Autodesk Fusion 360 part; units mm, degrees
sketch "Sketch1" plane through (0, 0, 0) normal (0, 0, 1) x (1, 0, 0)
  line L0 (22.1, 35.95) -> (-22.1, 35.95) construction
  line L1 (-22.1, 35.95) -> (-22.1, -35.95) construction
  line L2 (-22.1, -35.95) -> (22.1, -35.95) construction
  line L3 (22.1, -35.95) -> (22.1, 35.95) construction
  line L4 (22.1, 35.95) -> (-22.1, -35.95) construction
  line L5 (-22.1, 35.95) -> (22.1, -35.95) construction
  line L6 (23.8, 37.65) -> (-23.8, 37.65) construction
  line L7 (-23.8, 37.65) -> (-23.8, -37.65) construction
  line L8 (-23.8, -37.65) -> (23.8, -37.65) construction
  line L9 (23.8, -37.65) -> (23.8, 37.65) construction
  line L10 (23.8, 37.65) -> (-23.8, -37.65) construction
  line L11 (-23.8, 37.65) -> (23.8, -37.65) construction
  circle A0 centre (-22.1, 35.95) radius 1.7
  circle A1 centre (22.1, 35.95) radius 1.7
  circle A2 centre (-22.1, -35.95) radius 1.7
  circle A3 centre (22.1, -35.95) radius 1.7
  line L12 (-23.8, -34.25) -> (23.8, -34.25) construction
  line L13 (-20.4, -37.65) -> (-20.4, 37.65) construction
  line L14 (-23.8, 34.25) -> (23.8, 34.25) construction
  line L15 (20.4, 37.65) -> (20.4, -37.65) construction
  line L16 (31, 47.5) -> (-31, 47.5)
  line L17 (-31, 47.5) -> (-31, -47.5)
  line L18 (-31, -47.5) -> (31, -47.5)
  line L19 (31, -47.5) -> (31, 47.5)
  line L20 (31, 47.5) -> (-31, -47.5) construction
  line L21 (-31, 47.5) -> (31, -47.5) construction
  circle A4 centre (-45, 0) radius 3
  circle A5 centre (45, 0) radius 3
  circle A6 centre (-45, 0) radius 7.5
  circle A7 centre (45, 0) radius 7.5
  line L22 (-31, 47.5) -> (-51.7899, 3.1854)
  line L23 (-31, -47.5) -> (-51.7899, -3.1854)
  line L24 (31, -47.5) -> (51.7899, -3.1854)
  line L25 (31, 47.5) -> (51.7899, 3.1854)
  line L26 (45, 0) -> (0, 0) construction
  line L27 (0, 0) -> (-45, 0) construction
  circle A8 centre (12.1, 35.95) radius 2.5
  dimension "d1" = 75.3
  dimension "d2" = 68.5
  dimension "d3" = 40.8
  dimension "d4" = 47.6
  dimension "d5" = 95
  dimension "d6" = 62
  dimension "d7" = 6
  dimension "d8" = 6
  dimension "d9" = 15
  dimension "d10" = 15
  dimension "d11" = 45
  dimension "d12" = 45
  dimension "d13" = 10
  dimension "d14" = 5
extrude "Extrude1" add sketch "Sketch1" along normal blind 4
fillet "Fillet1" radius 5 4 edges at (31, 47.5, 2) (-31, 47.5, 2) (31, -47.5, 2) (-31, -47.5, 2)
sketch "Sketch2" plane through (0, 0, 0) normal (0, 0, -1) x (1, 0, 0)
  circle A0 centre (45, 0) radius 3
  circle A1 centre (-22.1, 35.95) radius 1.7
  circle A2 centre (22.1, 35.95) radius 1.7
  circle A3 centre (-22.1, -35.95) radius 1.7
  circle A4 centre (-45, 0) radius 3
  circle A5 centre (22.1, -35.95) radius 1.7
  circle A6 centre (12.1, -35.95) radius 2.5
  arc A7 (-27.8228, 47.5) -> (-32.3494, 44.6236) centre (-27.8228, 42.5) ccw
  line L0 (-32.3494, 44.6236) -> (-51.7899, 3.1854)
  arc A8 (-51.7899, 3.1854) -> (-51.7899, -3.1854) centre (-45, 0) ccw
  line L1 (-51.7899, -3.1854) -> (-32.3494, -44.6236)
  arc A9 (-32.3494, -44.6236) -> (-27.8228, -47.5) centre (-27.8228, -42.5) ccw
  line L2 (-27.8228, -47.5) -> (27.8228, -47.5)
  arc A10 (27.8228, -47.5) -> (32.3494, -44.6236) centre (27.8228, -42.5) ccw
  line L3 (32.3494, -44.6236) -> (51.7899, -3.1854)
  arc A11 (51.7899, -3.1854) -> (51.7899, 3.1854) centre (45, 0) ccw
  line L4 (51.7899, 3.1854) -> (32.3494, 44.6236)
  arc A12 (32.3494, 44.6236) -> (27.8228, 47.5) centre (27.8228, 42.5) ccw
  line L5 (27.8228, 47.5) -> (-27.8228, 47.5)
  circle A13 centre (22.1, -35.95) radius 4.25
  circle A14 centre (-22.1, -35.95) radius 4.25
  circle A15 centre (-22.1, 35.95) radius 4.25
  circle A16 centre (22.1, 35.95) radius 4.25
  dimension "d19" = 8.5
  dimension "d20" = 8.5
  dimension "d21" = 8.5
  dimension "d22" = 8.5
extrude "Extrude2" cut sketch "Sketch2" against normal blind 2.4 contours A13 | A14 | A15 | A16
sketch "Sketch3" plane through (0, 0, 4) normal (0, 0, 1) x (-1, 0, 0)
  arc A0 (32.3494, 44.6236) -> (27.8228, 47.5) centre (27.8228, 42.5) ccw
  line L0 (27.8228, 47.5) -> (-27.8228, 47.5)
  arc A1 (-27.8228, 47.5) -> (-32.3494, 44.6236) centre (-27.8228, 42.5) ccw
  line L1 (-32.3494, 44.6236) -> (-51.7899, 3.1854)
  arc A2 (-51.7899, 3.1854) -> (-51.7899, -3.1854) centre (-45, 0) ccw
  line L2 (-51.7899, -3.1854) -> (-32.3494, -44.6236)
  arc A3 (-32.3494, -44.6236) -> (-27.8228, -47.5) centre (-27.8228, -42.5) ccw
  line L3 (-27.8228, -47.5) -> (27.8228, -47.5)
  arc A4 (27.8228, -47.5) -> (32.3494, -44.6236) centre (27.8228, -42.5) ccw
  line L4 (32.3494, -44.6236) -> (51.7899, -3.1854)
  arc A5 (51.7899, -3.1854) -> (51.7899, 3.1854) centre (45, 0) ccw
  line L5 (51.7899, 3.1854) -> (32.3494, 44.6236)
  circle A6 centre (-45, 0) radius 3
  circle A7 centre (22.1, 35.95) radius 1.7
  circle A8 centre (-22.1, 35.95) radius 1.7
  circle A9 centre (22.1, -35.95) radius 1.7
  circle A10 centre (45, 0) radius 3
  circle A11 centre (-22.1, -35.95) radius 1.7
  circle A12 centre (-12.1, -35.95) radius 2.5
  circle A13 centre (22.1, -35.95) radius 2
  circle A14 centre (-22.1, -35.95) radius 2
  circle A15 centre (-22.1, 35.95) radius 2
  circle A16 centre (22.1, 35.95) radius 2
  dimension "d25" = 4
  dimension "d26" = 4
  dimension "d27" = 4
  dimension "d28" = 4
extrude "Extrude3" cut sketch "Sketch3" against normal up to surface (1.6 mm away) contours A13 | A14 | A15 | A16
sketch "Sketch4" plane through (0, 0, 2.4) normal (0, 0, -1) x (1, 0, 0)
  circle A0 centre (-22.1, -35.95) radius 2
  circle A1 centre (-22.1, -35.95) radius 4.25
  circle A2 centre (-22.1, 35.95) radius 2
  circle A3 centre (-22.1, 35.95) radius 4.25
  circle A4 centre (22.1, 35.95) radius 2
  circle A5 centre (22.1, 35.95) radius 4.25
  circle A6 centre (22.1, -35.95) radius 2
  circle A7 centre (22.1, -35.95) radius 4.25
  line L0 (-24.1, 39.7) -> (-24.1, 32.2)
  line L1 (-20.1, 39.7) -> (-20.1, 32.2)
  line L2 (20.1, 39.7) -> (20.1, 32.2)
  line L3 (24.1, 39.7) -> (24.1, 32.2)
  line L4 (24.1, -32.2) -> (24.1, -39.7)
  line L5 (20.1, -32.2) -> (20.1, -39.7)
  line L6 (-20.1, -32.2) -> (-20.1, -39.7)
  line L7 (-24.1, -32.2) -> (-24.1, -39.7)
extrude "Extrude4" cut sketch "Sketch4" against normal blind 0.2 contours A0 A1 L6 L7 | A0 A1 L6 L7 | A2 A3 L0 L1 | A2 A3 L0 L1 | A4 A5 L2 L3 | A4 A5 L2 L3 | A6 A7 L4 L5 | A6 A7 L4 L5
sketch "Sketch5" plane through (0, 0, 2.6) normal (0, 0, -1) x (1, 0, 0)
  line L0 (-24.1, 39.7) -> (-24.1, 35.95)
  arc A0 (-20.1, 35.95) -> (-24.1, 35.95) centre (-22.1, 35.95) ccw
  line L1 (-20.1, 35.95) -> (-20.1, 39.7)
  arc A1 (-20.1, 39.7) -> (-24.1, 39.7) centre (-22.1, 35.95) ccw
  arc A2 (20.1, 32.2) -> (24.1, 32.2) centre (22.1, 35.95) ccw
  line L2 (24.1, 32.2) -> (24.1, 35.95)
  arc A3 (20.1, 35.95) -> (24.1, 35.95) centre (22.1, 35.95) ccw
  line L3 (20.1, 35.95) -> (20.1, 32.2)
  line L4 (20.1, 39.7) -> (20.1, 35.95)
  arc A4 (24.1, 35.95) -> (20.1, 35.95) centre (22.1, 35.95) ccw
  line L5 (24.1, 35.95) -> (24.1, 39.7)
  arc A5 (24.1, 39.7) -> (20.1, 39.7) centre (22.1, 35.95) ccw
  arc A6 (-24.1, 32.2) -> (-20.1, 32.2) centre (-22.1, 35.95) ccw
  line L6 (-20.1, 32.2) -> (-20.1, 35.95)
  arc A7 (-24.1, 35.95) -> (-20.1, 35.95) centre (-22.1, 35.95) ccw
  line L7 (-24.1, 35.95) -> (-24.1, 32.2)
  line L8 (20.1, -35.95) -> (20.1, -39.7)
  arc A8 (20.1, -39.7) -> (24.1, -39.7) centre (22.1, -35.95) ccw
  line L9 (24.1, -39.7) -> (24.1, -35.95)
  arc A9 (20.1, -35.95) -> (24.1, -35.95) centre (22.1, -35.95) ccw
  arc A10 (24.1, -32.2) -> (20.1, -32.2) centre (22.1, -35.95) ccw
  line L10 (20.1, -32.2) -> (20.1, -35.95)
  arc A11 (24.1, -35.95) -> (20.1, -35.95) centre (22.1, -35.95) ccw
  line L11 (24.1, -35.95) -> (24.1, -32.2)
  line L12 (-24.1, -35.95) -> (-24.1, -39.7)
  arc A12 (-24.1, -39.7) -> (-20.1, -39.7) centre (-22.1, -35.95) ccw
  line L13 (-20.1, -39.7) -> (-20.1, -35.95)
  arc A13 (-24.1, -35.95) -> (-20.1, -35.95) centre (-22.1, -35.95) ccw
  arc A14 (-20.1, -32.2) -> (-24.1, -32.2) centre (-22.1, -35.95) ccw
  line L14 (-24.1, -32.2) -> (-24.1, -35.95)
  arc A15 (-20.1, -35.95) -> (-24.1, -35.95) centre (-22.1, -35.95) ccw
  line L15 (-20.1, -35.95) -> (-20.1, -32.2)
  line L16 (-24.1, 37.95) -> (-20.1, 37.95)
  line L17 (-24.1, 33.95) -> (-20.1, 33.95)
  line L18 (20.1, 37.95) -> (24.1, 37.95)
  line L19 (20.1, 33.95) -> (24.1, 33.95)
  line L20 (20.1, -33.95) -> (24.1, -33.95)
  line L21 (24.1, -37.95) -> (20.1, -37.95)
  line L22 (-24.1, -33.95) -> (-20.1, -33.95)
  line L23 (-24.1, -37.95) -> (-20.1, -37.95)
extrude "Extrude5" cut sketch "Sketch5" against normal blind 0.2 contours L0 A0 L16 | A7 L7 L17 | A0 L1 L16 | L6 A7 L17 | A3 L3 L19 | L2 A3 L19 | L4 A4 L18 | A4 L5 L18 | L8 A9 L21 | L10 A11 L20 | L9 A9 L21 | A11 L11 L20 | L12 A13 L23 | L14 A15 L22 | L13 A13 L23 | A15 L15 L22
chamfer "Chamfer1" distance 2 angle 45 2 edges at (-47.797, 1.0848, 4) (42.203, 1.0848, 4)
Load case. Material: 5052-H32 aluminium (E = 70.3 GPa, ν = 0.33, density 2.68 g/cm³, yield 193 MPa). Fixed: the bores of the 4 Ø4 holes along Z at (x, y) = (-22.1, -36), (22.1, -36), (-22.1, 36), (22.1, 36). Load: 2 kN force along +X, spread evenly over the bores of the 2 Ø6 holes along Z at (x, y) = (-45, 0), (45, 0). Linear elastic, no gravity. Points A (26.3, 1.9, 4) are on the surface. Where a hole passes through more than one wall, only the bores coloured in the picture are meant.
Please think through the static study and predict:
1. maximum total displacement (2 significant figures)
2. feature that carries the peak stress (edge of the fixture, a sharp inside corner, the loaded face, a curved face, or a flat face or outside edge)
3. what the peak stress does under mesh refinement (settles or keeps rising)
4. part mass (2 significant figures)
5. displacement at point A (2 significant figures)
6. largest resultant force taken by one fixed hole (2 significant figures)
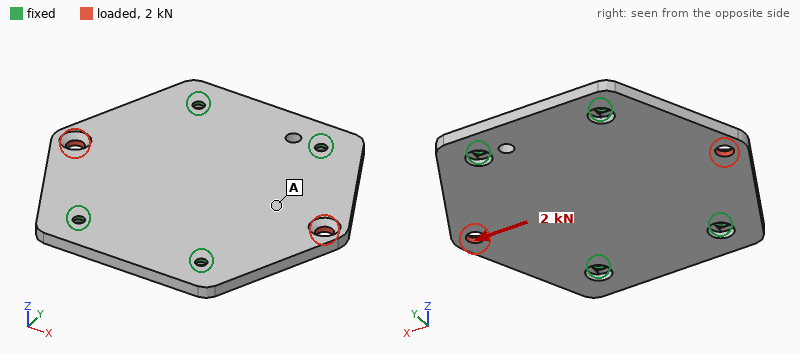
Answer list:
54 µm
edge of the fixture
keeps rising
83 g
11 µm
520 N
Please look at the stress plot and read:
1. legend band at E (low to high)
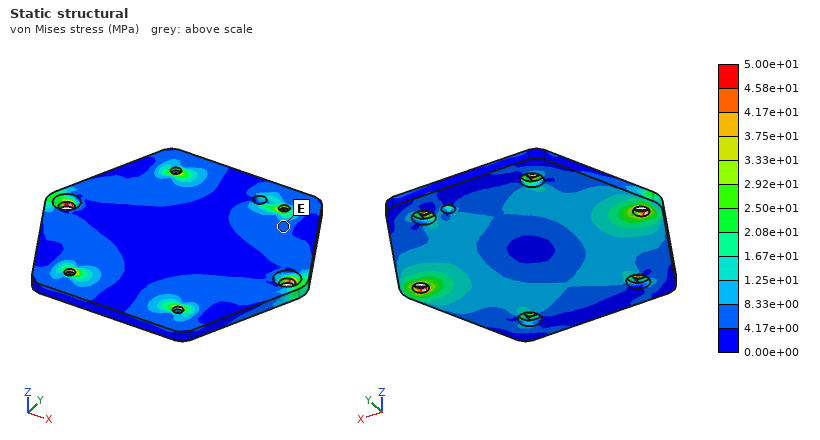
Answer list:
4.17e+00 to 8.33e+00 MPa
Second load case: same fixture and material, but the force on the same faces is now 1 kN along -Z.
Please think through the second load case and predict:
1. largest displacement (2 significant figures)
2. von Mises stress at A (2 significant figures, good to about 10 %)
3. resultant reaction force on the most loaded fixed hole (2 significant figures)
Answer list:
0.47 mm
55 MPa
1.3 kN
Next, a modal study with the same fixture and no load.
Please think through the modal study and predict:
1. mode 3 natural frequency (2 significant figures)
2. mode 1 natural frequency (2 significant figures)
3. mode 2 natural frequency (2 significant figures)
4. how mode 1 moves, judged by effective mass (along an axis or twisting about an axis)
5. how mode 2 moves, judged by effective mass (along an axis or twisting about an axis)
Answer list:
3800 Hz
2300 Hz
2400 Hz
along Z
twisting about Y
